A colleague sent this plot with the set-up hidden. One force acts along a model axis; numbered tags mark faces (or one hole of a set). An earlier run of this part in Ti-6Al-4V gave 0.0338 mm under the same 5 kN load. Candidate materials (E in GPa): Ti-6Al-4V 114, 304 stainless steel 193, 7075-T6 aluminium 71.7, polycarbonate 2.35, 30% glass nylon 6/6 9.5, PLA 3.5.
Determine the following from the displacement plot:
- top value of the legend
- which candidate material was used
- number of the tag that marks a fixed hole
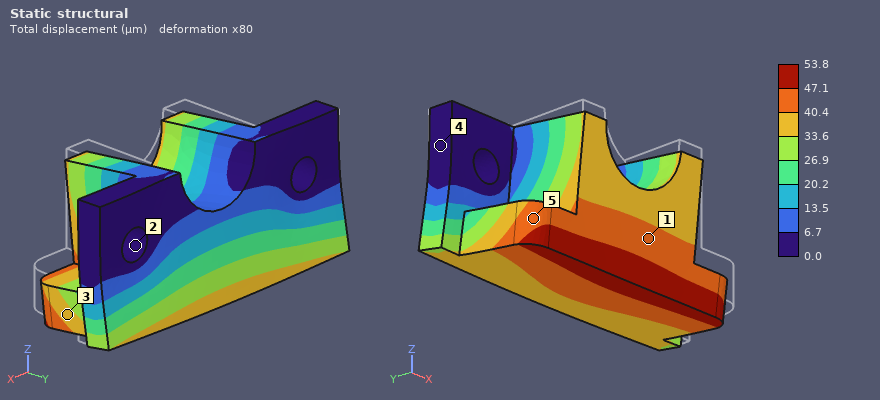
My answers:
53.8 µm
7075-T6 aluminium
2
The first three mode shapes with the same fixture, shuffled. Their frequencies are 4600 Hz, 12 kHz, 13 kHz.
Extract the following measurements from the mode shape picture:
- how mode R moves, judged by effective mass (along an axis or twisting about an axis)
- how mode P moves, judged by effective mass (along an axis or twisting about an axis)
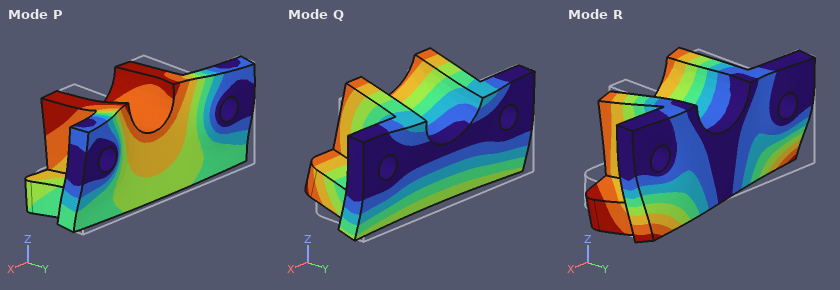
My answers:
along X
along Y
